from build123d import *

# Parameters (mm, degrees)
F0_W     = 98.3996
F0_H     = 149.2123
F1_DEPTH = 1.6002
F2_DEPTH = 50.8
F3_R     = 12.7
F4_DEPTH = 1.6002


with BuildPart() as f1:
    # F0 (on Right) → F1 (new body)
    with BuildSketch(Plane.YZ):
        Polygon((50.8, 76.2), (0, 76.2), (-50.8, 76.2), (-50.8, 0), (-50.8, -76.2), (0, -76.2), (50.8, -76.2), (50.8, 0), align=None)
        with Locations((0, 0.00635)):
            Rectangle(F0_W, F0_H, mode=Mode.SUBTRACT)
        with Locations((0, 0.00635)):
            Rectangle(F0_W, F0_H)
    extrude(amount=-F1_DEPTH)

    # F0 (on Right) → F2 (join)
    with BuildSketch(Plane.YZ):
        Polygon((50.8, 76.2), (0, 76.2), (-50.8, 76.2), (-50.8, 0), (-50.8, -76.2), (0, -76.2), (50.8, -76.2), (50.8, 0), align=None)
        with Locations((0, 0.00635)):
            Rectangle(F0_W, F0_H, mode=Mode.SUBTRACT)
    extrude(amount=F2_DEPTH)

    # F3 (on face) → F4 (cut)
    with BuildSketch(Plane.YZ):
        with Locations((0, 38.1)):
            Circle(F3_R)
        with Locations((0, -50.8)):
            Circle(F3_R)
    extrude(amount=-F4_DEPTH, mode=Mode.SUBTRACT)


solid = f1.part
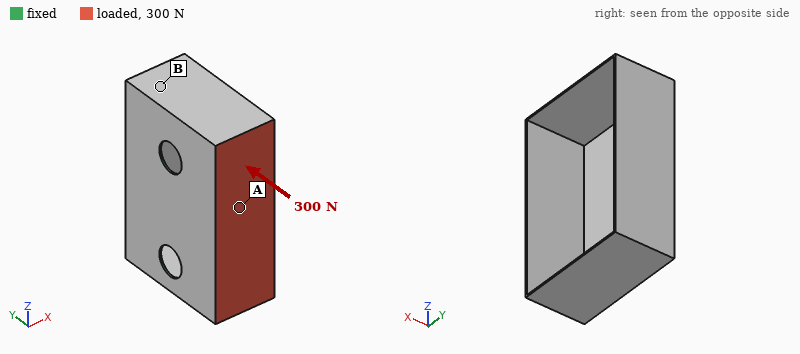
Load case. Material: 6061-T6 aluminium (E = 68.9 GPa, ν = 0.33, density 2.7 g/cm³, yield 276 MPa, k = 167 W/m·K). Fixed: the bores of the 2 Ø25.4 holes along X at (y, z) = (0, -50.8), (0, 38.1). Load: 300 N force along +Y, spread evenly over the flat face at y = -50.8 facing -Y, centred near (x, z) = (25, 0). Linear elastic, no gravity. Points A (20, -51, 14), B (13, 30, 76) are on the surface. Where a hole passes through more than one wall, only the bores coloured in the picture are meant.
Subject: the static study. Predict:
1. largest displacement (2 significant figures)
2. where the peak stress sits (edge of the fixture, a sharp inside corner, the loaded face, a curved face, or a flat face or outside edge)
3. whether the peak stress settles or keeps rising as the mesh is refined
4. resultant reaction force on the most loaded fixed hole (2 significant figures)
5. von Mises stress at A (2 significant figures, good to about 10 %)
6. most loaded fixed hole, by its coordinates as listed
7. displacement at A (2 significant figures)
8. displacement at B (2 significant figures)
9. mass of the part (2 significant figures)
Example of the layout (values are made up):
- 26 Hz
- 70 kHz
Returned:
- 1.8 mm
- edge of the fixture
- keeps rising
- 180 N
- 16 MPa
- (0, 38.1)
- 0.77 mm
- 0.27 mm
- 170 g
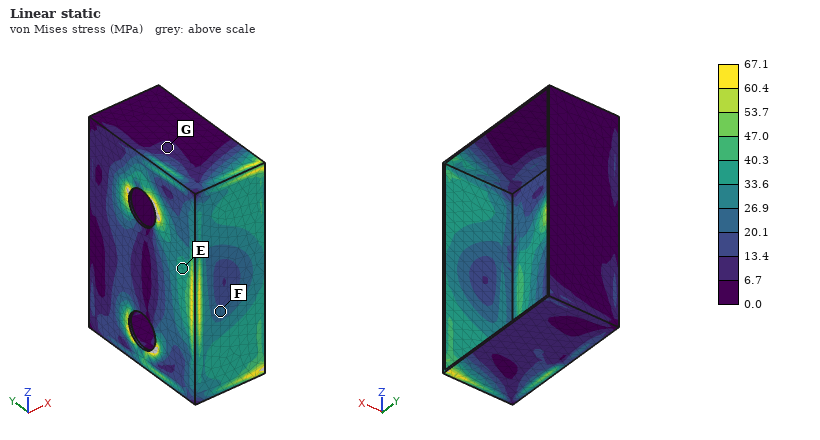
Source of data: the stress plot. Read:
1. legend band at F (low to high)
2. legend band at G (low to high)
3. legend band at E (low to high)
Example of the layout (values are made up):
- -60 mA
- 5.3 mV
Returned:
- 20.1 to 26.9 MPa
- 6.7 to 13.4 MPa
- 33.6 to 40.3 MPa
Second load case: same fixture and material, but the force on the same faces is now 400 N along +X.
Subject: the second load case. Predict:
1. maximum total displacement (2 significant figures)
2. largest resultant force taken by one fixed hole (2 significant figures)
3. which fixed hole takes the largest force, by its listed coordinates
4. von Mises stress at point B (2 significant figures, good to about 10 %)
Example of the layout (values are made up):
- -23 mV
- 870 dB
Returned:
- 1.8 mm
- 220 N
- (0, 38.1)
- 12 MPa
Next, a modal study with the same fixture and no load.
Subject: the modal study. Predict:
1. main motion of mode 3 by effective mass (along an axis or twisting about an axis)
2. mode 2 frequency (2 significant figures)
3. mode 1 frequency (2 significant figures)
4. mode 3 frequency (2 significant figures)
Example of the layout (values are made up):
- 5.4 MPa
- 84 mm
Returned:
- along X
- 350 Hz
- 270 Hz
- 480 Hz
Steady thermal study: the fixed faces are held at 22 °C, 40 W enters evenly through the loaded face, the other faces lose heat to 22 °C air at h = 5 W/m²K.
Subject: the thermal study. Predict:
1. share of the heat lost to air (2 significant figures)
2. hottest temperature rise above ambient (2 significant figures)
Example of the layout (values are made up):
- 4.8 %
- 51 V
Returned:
- 13 %
- 51 K
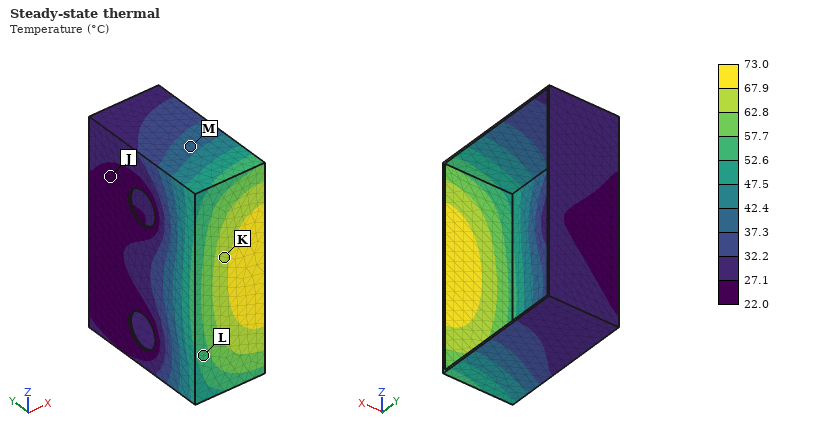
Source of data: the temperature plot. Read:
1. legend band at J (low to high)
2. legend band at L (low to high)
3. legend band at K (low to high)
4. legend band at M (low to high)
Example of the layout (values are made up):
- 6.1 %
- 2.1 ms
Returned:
- 22.0 to 27.1 °C
- 52.6 to 57.7 °C
- 62.8 to 67.9 °C
- 37.3 to 42.4 °C
